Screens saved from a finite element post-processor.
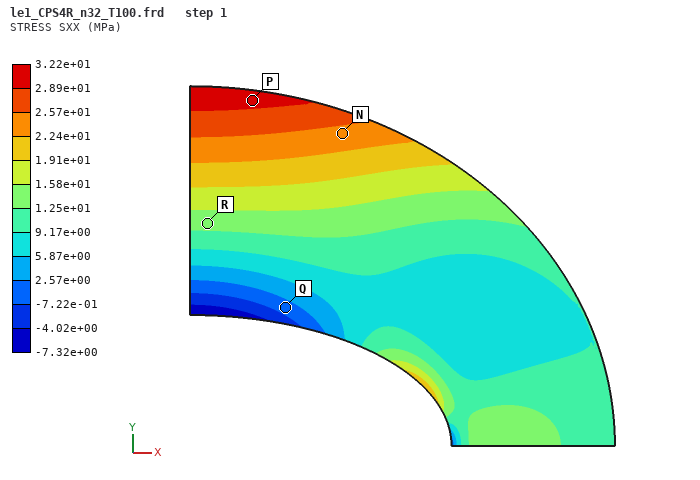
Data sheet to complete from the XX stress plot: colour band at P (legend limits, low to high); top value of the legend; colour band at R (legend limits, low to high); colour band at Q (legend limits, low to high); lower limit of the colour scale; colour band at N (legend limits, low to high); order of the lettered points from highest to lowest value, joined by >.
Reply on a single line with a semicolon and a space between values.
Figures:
2.89e+01 to 3.22e+01 MPa; 3.22e+01 MPa; 1.25e+01 to 1.58e+01 MPa; -7.22e-01 to 2.57e+00 MPa; -7.32e+00 MPa; 2.24e+01 to 2.57e+01 MPa; P > N > R > Q
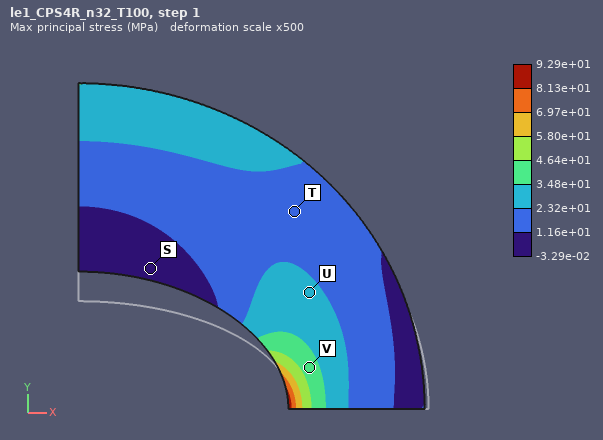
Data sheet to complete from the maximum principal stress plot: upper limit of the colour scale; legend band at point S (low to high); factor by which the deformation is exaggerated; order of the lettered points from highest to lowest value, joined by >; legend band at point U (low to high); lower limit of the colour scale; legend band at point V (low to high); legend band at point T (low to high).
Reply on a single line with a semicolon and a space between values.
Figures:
9.29e+01 MPa; -3.29e-02 to 1.16e+01 MPa; 500; V > U > T > S; 2.32e+01 to 3.48e+01 MPa; -3.29e-02 MPa; 3.48e+01 to 4.64e+01 MPa; 1.16e+01 to 2.32e+01 MPa
